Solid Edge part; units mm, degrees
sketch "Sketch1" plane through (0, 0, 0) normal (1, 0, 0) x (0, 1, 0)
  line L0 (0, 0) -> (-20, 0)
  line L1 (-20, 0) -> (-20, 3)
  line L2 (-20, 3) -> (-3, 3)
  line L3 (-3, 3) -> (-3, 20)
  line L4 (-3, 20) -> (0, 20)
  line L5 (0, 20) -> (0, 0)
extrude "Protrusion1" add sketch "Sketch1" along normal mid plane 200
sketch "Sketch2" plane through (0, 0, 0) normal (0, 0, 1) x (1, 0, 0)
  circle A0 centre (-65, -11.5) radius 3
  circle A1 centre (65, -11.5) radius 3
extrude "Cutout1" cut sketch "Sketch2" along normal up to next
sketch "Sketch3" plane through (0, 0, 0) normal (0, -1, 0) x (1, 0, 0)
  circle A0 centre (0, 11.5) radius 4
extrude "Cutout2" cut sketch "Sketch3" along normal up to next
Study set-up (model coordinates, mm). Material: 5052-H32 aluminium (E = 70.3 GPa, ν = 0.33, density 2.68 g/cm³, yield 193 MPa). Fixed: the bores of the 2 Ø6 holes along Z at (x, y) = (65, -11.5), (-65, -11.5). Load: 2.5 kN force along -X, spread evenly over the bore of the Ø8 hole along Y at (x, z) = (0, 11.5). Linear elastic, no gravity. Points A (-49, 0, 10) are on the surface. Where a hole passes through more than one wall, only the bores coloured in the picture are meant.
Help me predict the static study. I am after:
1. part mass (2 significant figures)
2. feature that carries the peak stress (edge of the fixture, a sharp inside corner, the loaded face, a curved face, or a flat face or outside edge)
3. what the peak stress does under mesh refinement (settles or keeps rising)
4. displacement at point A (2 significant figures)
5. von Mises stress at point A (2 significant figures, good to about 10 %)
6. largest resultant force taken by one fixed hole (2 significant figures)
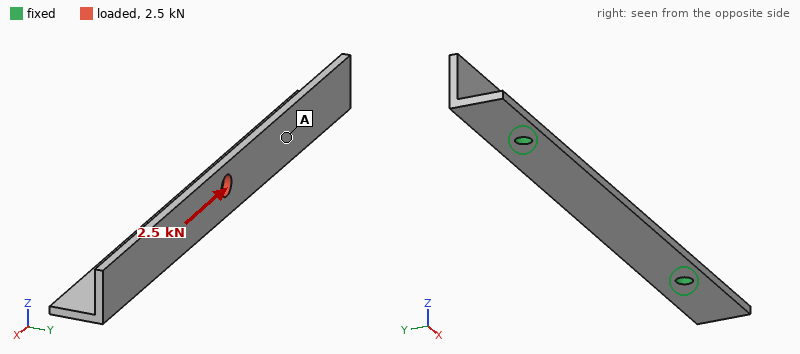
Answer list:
59 g
edge of the fixture
keeps rising
15 µm
8.4 MPa
1.3 kN
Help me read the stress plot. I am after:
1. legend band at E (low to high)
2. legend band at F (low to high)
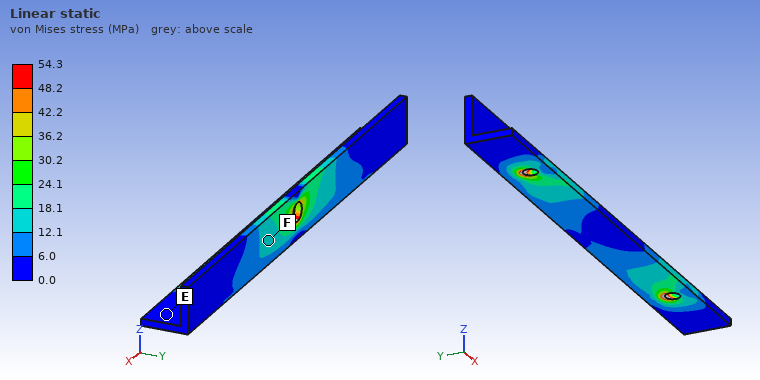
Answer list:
0.0 to 6.0 MPa
12.1 to 18.1 MPa
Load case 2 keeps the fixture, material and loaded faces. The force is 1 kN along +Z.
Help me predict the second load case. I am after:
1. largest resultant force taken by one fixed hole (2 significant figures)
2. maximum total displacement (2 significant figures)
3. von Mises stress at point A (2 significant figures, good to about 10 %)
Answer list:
940 N
0.26 mm
27 MPa
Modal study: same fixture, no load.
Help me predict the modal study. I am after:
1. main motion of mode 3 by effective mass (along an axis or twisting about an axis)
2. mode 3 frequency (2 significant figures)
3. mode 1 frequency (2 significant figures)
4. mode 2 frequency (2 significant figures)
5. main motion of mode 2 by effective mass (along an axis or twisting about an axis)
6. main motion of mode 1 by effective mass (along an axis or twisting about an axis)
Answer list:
twisting about Z
3200 Hz
2000 Hz
2400 Hz
along Z
along Y
